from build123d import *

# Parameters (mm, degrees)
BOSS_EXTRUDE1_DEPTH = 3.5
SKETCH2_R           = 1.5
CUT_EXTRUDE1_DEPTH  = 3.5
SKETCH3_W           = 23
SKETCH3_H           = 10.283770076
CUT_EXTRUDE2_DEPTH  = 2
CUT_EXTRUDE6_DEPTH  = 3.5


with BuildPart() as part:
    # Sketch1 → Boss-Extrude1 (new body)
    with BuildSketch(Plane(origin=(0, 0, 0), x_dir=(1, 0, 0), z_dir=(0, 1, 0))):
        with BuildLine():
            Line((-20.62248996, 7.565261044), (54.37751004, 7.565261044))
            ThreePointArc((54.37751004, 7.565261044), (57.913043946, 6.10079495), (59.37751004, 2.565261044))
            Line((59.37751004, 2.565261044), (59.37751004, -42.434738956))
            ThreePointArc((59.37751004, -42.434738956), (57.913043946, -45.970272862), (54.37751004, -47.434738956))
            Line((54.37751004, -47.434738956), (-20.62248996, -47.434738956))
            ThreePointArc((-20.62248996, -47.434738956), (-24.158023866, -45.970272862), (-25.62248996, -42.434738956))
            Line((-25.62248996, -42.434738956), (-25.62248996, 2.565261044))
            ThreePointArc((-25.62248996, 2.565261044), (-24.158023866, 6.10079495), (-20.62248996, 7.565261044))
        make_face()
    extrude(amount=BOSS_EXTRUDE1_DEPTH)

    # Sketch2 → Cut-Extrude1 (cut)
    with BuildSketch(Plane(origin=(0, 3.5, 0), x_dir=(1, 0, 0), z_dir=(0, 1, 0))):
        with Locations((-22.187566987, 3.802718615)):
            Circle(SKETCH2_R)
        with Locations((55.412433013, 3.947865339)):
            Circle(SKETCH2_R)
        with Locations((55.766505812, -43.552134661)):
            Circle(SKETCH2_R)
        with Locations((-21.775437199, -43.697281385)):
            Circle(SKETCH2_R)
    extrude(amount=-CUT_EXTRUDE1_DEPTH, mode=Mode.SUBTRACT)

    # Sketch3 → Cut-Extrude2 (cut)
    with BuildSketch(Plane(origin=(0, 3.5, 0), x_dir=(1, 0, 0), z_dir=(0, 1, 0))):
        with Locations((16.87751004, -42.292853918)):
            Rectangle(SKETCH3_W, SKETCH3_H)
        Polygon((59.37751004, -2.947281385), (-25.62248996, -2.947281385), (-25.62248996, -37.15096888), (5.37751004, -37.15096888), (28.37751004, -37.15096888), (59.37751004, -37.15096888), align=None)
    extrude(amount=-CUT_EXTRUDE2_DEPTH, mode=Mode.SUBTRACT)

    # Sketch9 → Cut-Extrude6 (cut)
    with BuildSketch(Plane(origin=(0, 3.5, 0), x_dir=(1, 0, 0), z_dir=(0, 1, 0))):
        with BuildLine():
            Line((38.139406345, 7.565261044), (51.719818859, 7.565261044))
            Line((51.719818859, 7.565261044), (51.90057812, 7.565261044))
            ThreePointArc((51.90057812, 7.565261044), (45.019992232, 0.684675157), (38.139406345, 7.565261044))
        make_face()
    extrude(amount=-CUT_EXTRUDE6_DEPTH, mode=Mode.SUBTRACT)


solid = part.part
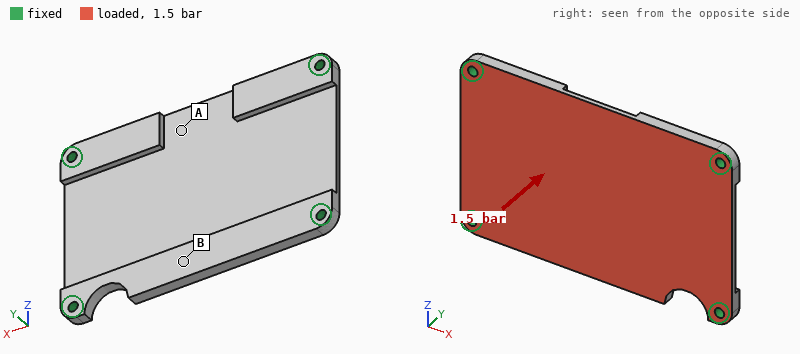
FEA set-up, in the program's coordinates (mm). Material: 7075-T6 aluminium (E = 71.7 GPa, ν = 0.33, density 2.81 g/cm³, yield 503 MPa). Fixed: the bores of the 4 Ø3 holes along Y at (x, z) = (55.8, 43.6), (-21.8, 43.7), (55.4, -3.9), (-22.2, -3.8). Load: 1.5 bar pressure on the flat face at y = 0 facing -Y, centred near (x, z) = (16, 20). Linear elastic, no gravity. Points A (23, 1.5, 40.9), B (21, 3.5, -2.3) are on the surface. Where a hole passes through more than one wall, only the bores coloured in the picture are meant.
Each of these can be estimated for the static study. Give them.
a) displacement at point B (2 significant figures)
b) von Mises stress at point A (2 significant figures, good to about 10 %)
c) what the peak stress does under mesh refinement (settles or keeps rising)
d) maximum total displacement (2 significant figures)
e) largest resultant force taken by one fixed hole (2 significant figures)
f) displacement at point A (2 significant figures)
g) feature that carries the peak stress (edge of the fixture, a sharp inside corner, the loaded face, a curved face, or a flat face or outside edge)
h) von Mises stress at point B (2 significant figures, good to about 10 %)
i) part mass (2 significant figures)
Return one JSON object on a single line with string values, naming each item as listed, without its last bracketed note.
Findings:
{"displacement at point B": "0.13 mm", "von Mises stress at point A": "16 MPa", "what the peak stress does under mesh refinement": "keeps rising", "maximum total displacement": "0.22 mm", "largest resultant force taken by one fixed hole": "510 N", "displacement at point A": "0.17 mm", "feature that carries the peak stress": "edge of the fixture", "von Mises stress at point B": "44 MPa", "part mass": "27 g"}
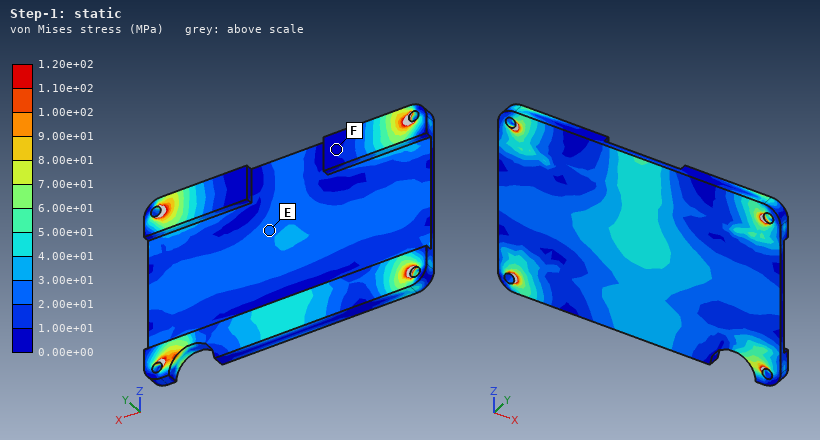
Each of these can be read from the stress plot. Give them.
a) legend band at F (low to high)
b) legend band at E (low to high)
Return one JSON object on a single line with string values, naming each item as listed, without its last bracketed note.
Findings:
{"legend band at F": "0.00e+00 to 1.00e+01 MPa", "legend band at E": "2.00e+01 to 3.00e+01 MPa"}
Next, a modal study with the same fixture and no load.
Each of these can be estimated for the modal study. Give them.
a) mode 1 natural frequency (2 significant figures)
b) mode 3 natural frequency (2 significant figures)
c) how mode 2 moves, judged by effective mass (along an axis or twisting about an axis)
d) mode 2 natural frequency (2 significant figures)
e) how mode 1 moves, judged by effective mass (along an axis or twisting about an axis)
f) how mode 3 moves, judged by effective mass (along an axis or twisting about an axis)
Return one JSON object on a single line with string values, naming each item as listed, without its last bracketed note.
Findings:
{"mode 1 natural frequency": "2300 Hz", "mode 3 natural frequency": "4700 Hz", "how mode 2 moves, judged by effective mass": "twisting about X", "mode 2 natural frequency": "3100 Hz", "how mode 1 moves, judged by effective mass": "along Y", "how mode 3 moves, judged by effective mass": "twisting about Z"}
